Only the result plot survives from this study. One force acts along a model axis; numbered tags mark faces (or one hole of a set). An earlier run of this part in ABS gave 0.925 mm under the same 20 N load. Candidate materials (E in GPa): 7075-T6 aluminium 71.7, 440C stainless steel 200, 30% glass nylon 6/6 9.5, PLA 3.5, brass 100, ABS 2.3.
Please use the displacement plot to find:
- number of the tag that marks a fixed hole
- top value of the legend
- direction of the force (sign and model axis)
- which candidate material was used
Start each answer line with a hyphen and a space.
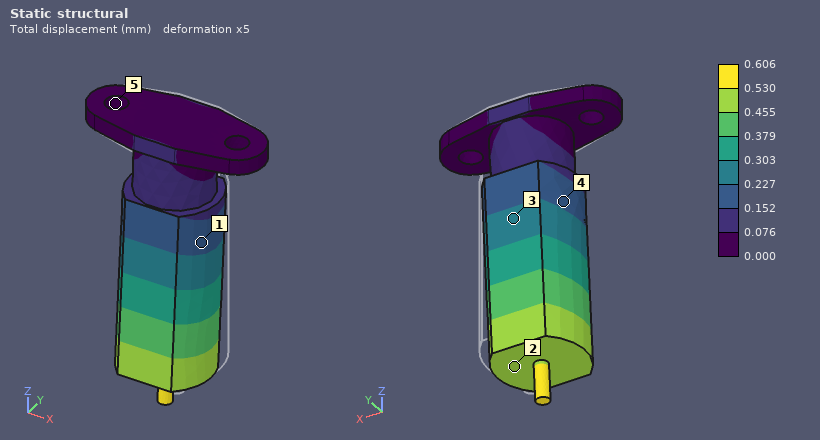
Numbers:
- 5
- 0.606 mm
- -Y
- PLA
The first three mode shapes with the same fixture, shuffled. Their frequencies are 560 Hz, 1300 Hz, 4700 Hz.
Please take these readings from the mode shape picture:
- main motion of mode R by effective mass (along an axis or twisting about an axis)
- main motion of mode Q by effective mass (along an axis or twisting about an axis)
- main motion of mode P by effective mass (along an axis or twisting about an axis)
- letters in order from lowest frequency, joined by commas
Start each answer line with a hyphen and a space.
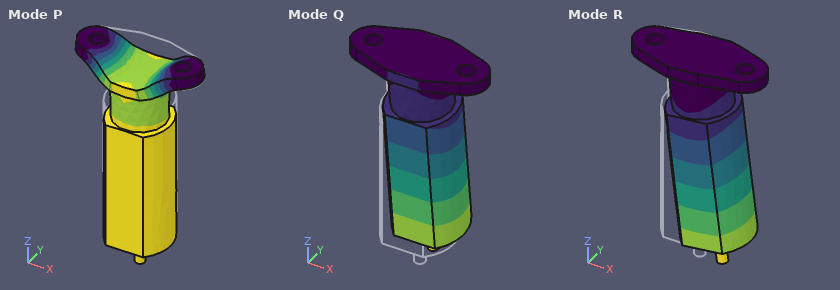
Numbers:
- along X
- along Y
- along Z
- Q, R, P
